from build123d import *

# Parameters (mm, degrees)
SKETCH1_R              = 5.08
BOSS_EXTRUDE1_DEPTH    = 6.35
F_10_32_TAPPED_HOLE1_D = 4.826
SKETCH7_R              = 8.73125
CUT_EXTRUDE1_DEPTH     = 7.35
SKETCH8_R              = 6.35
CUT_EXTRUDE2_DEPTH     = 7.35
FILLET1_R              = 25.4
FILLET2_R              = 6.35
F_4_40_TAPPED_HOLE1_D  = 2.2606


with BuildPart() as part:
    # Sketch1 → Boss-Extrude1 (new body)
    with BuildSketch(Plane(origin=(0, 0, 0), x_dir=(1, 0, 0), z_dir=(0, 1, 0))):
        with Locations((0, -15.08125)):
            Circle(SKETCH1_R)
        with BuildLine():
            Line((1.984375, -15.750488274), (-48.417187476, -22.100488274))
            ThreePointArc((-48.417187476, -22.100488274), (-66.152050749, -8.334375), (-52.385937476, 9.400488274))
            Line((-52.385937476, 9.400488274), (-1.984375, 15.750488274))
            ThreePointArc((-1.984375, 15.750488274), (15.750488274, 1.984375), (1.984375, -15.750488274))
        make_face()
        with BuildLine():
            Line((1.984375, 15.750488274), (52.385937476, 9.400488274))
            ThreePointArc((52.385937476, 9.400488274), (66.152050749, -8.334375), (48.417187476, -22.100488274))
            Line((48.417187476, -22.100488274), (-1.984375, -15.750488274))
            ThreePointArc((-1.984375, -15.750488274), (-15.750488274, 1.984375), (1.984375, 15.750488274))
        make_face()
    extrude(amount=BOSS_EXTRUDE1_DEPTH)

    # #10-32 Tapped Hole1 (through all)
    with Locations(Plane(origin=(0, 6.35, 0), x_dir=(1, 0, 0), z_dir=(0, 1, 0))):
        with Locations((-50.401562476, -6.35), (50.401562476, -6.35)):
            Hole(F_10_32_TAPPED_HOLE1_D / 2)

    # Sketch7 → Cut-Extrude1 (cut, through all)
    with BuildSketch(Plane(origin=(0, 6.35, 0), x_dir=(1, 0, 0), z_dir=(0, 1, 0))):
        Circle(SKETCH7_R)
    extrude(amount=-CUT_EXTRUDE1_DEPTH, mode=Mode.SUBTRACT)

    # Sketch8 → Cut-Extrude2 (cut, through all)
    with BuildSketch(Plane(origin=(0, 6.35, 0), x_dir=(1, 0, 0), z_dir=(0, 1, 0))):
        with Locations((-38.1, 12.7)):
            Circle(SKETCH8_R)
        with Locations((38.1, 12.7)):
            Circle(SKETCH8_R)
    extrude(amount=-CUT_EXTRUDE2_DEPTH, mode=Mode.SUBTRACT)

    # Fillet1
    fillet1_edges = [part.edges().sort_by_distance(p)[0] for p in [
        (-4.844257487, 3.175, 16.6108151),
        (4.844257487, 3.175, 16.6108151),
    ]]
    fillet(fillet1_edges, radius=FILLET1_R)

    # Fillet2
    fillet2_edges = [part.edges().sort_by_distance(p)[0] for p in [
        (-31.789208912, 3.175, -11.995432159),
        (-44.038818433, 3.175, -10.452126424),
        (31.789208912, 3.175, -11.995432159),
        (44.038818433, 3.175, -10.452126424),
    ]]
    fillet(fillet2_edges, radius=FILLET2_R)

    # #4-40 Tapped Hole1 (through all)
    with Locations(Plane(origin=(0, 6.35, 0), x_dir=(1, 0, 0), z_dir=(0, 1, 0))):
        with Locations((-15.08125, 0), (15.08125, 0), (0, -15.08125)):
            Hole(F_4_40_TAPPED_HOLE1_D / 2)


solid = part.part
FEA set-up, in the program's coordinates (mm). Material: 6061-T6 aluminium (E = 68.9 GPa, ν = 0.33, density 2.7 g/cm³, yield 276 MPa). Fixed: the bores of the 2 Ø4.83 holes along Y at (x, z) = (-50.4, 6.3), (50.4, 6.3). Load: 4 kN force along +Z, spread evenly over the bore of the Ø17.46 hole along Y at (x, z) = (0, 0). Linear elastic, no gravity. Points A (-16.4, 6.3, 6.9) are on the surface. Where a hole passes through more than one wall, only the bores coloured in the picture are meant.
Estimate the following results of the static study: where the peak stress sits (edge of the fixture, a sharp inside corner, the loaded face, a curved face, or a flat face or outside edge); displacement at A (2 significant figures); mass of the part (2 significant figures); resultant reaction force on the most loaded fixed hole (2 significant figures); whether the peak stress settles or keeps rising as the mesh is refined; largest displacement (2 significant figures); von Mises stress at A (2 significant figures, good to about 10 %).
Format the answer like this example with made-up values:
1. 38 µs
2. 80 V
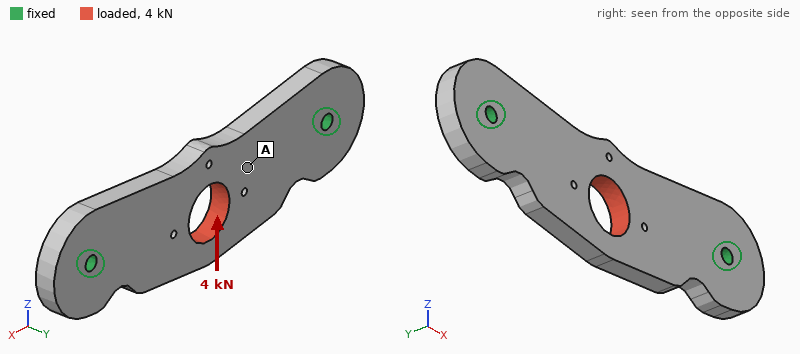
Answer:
1. edge of the fixture
2. 58 µm
3. 63 g
4. 2.2 kN
5. keeps rising
6. 72 µm
7. 18 MPa
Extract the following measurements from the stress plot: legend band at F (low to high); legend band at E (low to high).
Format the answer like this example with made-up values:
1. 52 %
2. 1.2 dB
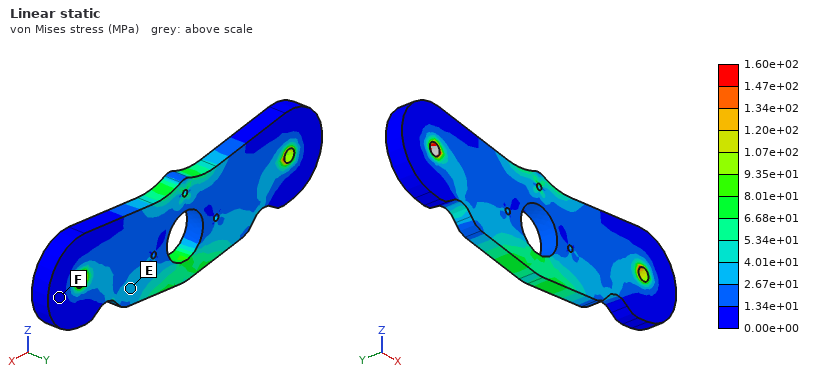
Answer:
1. 0.00e+00 to 1.34e+01 MPa
2. 2.67e+01 to 4.01e+01 MPa
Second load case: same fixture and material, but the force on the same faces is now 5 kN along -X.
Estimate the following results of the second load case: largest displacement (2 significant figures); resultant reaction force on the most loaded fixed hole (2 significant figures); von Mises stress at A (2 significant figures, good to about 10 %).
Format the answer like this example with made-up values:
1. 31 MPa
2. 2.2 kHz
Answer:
1. 14 µm
2. 2.5 kN
3. 13 MPa
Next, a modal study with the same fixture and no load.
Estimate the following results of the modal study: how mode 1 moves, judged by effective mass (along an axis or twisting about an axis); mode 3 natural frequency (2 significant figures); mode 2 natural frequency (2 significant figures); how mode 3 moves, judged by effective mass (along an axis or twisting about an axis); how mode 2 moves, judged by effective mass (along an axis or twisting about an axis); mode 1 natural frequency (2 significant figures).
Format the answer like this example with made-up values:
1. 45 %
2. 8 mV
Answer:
1. along Y
2. 7600 Hz
3. 5300 Hz
4. along Z
5. twisting about X
6. 2900 Hz
